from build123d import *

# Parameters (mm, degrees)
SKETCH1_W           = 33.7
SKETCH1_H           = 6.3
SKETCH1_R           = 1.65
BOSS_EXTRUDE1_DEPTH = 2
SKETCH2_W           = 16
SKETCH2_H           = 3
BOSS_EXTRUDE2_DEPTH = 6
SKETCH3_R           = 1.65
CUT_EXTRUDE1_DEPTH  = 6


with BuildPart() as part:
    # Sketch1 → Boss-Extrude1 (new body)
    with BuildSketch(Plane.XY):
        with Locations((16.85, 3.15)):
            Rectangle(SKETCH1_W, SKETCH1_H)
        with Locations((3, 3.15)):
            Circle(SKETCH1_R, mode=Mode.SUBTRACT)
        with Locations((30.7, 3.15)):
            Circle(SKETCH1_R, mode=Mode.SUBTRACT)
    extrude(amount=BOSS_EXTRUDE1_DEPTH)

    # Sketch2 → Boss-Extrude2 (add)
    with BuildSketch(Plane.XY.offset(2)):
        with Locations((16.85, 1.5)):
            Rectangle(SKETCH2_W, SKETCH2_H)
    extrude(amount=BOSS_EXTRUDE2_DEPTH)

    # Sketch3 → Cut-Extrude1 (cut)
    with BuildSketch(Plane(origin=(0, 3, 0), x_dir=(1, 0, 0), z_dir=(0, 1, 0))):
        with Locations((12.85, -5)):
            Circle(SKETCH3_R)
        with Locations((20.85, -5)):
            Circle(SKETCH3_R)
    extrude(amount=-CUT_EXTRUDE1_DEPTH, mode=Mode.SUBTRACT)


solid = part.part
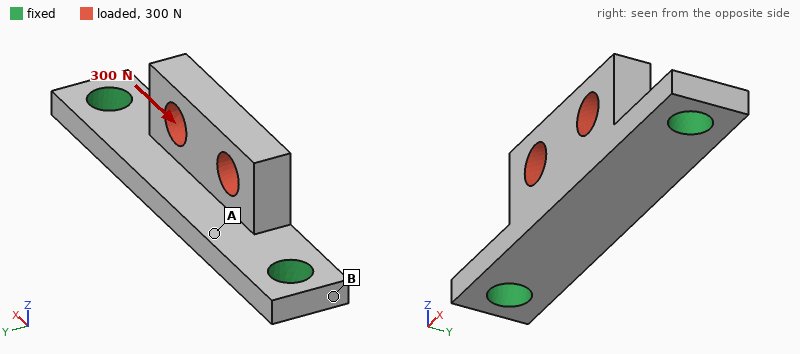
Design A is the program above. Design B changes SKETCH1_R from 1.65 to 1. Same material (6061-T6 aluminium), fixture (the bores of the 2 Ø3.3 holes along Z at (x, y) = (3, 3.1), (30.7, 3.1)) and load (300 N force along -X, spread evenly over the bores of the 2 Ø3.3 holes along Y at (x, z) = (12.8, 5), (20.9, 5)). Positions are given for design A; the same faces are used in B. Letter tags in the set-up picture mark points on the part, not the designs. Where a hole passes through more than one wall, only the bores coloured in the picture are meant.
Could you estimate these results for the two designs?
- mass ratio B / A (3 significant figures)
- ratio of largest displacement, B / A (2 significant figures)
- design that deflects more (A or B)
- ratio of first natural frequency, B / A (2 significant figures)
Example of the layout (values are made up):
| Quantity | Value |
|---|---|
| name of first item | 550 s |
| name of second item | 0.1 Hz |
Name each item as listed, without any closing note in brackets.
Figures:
| Quantity | Value |
|---|---|
| mass ratio B / A | 1.03 |
| ratio of largest displacement, B / A | 1.2 |
| design that deflects more | B |
| ratio of first natural frequency, B / A | 0.90 |
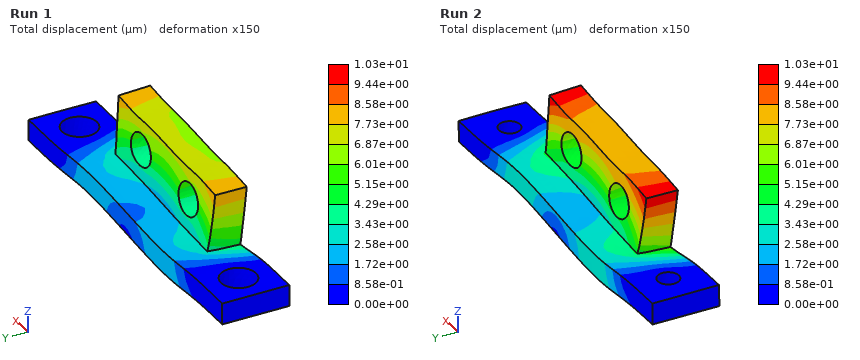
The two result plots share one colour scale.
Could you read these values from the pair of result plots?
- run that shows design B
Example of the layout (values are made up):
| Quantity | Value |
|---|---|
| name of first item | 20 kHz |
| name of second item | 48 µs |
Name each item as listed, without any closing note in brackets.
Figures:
| Quantity | Value |
|---|---|
| run that shows design B | Run 2 |
